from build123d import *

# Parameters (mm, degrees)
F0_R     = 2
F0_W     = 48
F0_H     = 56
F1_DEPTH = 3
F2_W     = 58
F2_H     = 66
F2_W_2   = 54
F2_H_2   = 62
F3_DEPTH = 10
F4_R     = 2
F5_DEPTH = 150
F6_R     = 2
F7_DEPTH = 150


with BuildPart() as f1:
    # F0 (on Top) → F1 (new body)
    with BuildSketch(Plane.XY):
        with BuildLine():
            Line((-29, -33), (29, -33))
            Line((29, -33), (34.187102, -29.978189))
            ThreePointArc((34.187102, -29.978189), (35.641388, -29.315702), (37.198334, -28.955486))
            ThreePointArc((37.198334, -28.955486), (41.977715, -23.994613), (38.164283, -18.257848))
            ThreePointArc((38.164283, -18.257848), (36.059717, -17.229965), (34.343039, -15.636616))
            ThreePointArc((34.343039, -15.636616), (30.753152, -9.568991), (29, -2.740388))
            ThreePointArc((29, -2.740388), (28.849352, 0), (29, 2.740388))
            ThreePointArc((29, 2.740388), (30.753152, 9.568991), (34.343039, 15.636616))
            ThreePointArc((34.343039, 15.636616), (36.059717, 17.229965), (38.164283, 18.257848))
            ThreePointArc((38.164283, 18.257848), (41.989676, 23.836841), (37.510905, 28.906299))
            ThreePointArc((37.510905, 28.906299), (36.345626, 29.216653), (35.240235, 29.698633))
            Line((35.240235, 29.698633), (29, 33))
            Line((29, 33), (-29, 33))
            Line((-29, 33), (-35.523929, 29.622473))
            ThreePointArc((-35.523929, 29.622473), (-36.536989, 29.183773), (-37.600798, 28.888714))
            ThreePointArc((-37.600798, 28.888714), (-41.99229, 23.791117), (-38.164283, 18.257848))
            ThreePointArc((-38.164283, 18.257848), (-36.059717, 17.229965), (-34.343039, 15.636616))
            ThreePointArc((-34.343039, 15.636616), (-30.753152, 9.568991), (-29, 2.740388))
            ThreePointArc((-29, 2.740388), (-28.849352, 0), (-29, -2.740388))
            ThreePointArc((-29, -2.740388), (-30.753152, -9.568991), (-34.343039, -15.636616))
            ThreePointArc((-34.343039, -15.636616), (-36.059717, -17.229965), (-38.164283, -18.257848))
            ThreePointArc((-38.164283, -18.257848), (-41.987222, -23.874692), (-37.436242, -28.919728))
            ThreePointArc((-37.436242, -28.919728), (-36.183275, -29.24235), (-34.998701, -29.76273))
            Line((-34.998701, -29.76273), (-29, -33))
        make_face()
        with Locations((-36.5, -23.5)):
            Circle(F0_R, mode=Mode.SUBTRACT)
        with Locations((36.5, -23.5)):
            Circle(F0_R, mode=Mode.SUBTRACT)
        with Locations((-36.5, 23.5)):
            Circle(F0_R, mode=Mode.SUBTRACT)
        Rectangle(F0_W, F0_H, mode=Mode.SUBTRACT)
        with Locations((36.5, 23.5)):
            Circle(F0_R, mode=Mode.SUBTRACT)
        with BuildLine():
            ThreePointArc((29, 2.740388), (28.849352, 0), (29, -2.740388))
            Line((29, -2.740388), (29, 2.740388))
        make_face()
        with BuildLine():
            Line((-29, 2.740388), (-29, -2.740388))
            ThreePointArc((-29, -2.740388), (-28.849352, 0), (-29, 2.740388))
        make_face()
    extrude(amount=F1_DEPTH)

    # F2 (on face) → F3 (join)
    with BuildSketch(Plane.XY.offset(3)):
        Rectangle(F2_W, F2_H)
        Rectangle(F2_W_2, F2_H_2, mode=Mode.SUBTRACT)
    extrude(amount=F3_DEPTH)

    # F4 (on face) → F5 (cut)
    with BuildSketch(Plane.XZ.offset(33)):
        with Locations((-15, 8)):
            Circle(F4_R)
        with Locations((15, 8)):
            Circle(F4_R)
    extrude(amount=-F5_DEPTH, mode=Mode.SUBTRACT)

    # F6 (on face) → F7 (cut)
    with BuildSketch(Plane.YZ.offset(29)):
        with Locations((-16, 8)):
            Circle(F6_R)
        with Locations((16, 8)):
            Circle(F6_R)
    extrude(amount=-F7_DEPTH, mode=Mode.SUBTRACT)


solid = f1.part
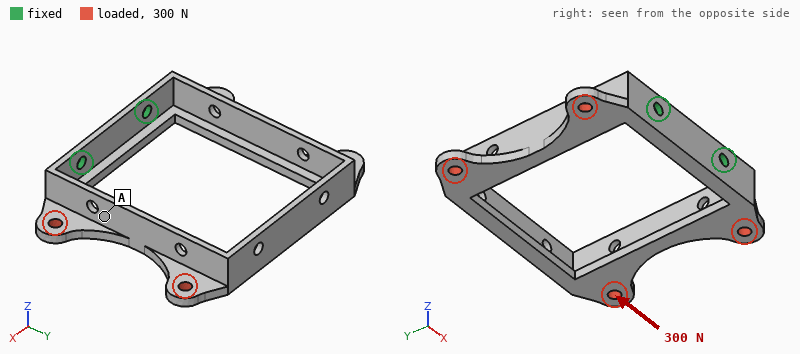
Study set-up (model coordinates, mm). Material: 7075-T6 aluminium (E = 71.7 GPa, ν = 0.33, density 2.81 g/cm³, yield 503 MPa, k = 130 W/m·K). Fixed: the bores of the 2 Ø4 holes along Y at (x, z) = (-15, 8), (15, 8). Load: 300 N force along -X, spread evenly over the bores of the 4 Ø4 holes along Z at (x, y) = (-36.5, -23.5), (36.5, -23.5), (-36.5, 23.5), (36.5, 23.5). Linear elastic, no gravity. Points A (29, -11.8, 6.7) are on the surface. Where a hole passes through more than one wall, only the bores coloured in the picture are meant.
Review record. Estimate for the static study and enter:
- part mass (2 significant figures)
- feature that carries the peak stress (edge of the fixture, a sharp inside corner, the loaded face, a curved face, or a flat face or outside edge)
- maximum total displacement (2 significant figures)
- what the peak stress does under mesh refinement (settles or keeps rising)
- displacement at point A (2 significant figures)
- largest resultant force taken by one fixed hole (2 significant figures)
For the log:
28 g
edge of the fixture
0.91 mm
keeps rising
0.32 mm
270 N
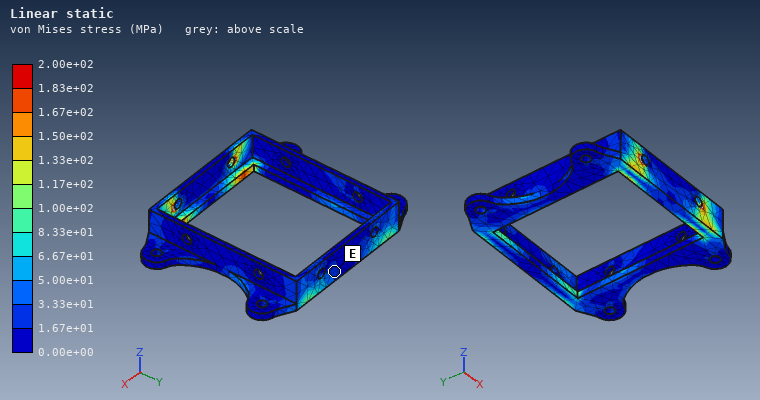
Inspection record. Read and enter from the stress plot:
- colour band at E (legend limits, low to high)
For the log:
1.67e+01 to 3.33e+01 MPa
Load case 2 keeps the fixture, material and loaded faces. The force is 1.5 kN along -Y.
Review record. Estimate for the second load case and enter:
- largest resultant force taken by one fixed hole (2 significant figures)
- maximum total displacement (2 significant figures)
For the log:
870 N
1.1 mm
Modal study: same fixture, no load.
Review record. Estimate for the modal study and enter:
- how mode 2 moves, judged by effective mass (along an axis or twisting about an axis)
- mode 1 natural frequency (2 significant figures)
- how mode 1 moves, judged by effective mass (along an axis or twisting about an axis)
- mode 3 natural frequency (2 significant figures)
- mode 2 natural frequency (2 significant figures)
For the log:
along X
410 Hz
along Z
830 Hz
570 Hz
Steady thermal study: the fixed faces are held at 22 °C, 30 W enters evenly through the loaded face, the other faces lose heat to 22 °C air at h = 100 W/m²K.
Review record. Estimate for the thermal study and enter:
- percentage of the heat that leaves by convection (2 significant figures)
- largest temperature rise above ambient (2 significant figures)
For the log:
68 %
42 K
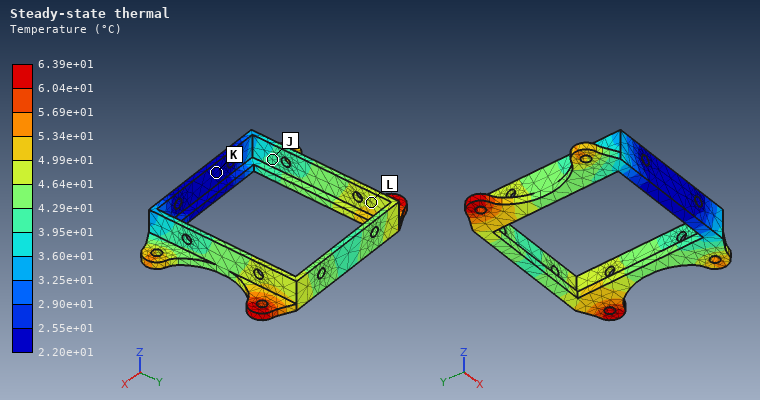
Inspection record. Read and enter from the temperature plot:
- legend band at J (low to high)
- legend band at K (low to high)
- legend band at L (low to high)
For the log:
3.95e+01 to 4.29e+01 °C
2.20e+01 to 2.55e+01 °C
4.64e+01 to 4.99e+01 °C
